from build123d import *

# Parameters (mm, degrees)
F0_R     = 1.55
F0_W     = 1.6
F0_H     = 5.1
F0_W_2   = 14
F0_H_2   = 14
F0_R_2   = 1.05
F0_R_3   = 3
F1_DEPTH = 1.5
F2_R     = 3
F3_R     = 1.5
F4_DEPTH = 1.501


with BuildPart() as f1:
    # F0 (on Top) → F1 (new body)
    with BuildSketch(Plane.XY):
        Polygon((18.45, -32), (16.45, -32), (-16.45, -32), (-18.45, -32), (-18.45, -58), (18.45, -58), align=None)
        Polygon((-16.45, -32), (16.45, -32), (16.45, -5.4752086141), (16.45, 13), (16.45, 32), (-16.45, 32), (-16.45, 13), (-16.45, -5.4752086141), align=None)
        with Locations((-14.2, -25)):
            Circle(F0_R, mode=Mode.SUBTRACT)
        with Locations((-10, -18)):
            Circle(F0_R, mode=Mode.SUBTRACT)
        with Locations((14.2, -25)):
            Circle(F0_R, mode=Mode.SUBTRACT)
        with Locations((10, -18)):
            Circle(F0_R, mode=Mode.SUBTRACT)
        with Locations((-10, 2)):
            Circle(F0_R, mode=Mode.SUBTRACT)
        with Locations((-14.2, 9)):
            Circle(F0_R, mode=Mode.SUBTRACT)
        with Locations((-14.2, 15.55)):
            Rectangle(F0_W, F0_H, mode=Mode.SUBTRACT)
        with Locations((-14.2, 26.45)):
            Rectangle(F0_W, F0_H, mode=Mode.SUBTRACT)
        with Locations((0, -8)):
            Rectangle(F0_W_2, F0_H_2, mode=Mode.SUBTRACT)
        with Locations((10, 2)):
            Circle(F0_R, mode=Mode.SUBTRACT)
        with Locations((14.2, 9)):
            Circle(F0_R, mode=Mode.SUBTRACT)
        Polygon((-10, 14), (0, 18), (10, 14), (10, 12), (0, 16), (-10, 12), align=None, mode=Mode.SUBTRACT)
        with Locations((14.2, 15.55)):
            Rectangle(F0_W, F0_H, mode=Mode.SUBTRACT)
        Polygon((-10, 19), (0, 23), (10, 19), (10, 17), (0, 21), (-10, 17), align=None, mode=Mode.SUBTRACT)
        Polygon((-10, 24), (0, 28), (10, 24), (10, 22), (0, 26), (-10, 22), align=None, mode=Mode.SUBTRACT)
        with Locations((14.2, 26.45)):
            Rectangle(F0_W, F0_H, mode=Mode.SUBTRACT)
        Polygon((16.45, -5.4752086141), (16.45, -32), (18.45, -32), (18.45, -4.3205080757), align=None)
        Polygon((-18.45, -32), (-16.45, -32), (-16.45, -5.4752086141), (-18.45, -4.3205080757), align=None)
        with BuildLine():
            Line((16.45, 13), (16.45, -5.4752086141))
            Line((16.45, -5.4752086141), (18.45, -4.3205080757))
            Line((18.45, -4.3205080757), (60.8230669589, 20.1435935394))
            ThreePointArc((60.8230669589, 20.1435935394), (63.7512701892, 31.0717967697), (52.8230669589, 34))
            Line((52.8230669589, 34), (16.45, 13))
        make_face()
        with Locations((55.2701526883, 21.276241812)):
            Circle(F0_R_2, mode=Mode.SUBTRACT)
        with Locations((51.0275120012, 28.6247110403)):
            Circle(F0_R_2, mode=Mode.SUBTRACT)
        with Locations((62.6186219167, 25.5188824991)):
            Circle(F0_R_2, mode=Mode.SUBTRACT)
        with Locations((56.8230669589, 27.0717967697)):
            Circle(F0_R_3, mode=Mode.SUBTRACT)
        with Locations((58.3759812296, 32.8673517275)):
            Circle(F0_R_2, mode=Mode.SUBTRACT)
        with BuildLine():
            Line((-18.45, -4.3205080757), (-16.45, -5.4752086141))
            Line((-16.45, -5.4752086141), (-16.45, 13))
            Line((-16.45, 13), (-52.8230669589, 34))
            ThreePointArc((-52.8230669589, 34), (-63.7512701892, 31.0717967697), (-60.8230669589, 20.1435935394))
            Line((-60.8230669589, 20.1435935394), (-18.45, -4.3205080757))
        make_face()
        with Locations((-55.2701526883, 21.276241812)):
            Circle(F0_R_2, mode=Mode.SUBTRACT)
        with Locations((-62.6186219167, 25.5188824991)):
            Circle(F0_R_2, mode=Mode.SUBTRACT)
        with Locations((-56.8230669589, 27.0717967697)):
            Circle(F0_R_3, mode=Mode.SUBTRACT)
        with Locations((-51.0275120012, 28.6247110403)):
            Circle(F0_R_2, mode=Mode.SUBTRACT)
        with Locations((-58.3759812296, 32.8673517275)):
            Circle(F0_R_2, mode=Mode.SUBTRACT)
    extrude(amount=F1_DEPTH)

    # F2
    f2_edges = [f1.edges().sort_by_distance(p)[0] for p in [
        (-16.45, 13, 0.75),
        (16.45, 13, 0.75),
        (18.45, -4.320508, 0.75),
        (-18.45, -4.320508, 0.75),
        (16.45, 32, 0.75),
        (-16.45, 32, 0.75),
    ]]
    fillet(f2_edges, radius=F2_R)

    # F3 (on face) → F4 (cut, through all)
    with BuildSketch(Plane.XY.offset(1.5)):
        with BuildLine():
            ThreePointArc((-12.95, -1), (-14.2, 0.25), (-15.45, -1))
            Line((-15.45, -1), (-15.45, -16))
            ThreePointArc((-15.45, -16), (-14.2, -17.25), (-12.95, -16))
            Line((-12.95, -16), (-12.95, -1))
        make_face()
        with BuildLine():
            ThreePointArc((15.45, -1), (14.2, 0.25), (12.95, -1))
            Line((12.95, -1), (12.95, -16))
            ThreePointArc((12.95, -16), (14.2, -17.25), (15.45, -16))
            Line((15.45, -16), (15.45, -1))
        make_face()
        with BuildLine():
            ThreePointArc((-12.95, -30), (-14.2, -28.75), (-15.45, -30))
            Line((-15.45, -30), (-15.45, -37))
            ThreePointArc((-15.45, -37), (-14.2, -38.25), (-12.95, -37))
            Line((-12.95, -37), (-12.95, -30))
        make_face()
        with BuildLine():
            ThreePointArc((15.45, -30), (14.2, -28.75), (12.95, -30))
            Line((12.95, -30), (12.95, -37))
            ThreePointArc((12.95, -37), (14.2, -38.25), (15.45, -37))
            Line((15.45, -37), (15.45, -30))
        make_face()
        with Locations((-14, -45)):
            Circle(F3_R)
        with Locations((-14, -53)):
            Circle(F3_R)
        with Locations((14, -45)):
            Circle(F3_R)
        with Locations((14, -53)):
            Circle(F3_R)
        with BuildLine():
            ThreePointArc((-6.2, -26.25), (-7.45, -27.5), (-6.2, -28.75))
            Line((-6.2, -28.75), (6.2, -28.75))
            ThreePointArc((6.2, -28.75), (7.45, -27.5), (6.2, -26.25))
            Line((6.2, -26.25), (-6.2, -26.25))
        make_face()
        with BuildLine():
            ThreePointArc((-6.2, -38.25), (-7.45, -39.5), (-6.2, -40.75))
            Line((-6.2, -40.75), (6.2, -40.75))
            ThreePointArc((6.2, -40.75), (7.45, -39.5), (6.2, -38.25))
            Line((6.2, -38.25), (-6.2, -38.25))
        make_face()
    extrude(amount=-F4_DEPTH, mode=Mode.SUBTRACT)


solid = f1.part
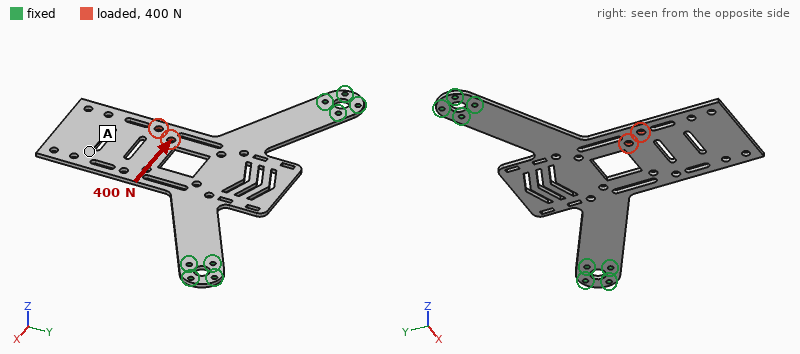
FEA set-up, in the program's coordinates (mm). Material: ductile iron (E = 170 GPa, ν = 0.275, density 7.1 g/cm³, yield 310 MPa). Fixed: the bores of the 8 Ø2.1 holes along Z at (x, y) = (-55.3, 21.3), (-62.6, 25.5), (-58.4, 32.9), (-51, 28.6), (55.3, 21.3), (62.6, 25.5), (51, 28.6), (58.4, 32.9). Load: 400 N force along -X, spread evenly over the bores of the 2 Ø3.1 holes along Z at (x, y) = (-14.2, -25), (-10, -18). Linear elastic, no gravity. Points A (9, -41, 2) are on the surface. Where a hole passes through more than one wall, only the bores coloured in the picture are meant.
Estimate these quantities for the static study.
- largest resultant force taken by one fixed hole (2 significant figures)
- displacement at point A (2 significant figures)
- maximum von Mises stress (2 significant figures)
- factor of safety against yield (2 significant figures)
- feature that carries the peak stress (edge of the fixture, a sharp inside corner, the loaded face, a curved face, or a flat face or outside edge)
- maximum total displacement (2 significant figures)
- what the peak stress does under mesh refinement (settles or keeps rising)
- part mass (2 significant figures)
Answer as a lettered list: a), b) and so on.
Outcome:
a) 230 N
b) 45 µm
c) 230 MPa
d) 1.4
e) a curved face
f) 52 µm
g) settles
h) 44 g
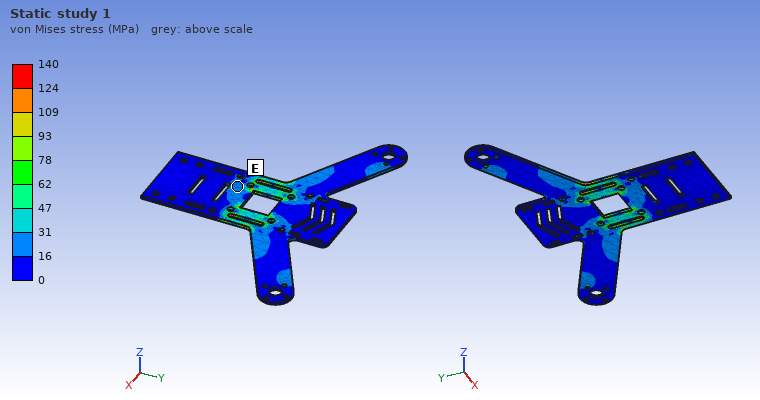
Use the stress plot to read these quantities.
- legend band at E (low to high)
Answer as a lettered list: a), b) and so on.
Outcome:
a) 16 to 31 MPa
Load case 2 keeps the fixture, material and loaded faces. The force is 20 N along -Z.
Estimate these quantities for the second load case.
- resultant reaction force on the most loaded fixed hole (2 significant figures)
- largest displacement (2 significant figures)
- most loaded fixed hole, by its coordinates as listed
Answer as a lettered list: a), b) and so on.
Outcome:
a) 41 N
b) 1.6 mm
c) (-55.3, 21.3)
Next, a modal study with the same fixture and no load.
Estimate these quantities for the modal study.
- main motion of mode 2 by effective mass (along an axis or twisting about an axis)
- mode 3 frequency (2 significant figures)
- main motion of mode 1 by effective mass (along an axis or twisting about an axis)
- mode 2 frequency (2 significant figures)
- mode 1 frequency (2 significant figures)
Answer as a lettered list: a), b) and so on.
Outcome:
a) along Z
b) 770 Hz
c) along Z
d) 510 Hz
e) 130 Hz
